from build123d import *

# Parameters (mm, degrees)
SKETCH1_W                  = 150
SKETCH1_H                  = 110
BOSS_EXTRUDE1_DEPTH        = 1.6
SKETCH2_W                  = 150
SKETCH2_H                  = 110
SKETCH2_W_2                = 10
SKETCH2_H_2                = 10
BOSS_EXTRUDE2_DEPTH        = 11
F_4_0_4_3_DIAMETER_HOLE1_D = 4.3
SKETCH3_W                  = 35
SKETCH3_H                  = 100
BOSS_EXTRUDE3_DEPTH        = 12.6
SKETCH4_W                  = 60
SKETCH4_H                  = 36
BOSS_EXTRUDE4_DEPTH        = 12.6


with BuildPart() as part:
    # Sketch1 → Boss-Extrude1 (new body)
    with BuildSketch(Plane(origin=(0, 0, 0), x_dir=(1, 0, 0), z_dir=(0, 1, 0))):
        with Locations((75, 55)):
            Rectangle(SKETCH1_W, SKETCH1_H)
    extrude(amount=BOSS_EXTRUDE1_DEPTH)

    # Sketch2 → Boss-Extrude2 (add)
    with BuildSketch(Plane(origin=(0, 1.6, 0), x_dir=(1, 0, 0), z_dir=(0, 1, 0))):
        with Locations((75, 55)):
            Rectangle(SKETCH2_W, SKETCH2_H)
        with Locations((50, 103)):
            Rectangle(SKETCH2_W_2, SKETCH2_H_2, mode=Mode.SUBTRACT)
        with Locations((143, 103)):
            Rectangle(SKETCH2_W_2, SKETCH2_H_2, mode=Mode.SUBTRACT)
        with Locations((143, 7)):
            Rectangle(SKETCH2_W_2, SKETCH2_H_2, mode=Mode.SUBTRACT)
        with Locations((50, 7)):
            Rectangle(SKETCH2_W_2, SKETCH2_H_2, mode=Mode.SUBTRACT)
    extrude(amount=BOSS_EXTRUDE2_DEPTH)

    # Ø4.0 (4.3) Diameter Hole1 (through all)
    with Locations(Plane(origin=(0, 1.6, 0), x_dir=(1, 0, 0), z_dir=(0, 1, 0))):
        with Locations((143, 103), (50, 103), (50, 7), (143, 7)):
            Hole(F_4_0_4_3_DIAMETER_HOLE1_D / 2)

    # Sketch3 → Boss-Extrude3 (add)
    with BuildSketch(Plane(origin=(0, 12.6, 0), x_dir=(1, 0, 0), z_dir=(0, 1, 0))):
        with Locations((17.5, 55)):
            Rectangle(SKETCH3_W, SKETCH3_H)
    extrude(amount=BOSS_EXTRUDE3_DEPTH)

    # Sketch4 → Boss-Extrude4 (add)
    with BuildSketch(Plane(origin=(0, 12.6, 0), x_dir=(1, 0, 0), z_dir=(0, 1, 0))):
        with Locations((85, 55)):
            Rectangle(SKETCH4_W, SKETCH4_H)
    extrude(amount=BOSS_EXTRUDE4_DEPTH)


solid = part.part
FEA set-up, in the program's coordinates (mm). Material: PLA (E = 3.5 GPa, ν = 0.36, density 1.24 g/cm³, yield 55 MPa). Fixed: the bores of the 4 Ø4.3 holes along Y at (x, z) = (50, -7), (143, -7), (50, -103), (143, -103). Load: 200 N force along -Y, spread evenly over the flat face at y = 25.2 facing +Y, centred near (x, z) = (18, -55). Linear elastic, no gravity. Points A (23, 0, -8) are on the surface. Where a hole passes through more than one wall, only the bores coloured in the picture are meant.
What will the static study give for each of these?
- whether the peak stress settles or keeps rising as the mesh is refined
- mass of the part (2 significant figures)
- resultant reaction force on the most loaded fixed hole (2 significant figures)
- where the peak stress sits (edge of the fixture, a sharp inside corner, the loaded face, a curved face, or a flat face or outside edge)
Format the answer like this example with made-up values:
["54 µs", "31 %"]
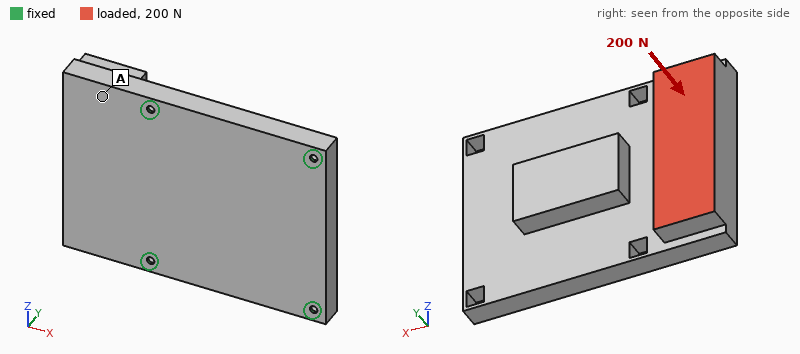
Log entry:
["keeps rising", "340 g", "170 N", "edge of the fixture"]
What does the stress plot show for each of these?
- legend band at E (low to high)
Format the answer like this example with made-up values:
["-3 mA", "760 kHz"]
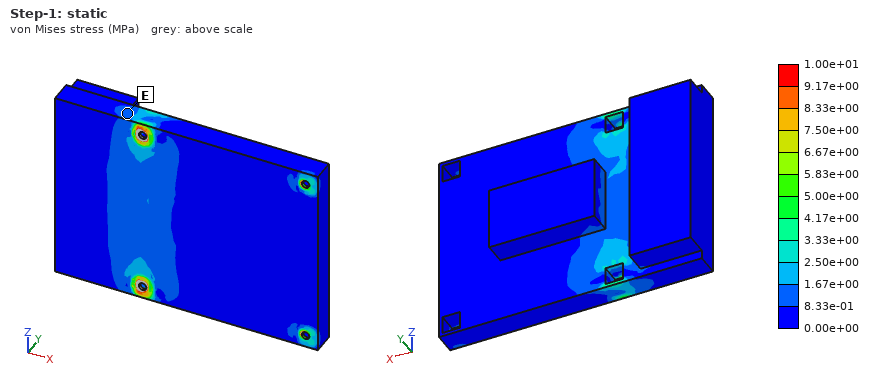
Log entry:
["8.33e-01 to 1.67e+00 MPa"]
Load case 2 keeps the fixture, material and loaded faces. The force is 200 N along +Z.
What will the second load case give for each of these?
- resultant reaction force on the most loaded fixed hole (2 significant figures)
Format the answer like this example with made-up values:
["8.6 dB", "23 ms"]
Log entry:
["120 N"]
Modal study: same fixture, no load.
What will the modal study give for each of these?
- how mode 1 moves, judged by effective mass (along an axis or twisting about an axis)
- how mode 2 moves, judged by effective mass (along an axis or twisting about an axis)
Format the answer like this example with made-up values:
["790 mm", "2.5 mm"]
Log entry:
["along Y", "along Y"]
